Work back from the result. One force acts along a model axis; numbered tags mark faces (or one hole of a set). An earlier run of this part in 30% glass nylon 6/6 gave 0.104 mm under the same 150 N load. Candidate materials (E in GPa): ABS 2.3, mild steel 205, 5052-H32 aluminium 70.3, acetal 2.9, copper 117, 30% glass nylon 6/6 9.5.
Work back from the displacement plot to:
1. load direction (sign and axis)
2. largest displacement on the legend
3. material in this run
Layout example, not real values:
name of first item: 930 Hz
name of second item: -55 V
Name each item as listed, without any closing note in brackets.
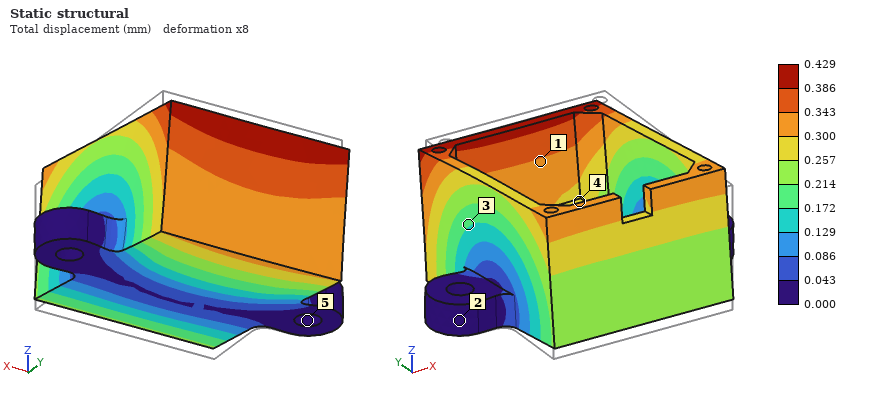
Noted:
load direction: -Z
largest displacement on the legend: 0.429 mm
material in this run: ABS
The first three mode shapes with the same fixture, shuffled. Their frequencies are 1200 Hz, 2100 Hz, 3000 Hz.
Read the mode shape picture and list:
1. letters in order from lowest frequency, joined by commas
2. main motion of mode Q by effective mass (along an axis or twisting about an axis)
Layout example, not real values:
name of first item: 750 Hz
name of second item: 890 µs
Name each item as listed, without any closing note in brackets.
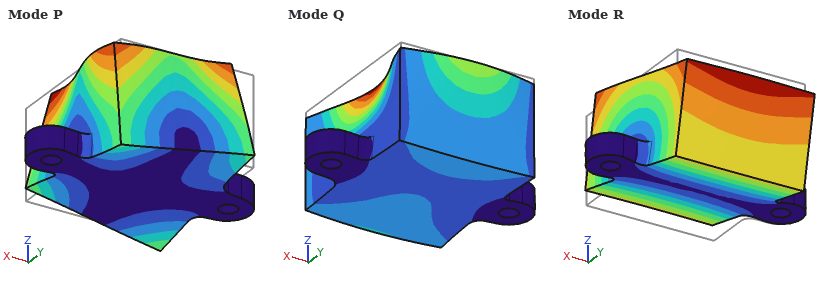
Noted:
letters in order from lowest frequency, joined by commas: R, P, Q
main motion of mode Q by effective mass: along Z
